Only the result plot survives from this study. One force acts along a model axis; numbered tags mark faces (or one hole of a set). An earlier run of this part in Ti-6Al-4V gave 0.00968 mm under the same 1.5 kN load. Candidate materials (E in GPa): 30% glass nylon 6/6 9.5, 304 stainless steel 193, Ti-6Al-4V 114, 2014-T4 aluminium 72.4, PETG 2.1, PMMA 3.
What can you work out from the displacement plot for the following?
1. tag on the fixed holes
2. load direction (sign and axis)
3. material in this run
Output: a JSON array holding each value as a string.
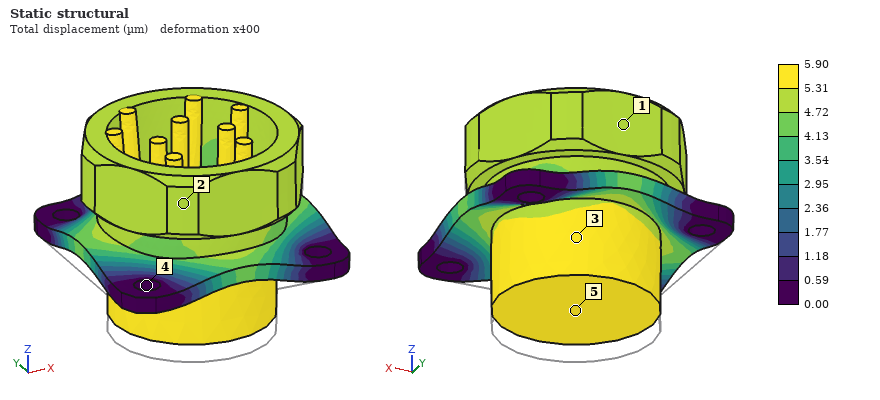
["4", "+Z", "304 stainless steel"]
